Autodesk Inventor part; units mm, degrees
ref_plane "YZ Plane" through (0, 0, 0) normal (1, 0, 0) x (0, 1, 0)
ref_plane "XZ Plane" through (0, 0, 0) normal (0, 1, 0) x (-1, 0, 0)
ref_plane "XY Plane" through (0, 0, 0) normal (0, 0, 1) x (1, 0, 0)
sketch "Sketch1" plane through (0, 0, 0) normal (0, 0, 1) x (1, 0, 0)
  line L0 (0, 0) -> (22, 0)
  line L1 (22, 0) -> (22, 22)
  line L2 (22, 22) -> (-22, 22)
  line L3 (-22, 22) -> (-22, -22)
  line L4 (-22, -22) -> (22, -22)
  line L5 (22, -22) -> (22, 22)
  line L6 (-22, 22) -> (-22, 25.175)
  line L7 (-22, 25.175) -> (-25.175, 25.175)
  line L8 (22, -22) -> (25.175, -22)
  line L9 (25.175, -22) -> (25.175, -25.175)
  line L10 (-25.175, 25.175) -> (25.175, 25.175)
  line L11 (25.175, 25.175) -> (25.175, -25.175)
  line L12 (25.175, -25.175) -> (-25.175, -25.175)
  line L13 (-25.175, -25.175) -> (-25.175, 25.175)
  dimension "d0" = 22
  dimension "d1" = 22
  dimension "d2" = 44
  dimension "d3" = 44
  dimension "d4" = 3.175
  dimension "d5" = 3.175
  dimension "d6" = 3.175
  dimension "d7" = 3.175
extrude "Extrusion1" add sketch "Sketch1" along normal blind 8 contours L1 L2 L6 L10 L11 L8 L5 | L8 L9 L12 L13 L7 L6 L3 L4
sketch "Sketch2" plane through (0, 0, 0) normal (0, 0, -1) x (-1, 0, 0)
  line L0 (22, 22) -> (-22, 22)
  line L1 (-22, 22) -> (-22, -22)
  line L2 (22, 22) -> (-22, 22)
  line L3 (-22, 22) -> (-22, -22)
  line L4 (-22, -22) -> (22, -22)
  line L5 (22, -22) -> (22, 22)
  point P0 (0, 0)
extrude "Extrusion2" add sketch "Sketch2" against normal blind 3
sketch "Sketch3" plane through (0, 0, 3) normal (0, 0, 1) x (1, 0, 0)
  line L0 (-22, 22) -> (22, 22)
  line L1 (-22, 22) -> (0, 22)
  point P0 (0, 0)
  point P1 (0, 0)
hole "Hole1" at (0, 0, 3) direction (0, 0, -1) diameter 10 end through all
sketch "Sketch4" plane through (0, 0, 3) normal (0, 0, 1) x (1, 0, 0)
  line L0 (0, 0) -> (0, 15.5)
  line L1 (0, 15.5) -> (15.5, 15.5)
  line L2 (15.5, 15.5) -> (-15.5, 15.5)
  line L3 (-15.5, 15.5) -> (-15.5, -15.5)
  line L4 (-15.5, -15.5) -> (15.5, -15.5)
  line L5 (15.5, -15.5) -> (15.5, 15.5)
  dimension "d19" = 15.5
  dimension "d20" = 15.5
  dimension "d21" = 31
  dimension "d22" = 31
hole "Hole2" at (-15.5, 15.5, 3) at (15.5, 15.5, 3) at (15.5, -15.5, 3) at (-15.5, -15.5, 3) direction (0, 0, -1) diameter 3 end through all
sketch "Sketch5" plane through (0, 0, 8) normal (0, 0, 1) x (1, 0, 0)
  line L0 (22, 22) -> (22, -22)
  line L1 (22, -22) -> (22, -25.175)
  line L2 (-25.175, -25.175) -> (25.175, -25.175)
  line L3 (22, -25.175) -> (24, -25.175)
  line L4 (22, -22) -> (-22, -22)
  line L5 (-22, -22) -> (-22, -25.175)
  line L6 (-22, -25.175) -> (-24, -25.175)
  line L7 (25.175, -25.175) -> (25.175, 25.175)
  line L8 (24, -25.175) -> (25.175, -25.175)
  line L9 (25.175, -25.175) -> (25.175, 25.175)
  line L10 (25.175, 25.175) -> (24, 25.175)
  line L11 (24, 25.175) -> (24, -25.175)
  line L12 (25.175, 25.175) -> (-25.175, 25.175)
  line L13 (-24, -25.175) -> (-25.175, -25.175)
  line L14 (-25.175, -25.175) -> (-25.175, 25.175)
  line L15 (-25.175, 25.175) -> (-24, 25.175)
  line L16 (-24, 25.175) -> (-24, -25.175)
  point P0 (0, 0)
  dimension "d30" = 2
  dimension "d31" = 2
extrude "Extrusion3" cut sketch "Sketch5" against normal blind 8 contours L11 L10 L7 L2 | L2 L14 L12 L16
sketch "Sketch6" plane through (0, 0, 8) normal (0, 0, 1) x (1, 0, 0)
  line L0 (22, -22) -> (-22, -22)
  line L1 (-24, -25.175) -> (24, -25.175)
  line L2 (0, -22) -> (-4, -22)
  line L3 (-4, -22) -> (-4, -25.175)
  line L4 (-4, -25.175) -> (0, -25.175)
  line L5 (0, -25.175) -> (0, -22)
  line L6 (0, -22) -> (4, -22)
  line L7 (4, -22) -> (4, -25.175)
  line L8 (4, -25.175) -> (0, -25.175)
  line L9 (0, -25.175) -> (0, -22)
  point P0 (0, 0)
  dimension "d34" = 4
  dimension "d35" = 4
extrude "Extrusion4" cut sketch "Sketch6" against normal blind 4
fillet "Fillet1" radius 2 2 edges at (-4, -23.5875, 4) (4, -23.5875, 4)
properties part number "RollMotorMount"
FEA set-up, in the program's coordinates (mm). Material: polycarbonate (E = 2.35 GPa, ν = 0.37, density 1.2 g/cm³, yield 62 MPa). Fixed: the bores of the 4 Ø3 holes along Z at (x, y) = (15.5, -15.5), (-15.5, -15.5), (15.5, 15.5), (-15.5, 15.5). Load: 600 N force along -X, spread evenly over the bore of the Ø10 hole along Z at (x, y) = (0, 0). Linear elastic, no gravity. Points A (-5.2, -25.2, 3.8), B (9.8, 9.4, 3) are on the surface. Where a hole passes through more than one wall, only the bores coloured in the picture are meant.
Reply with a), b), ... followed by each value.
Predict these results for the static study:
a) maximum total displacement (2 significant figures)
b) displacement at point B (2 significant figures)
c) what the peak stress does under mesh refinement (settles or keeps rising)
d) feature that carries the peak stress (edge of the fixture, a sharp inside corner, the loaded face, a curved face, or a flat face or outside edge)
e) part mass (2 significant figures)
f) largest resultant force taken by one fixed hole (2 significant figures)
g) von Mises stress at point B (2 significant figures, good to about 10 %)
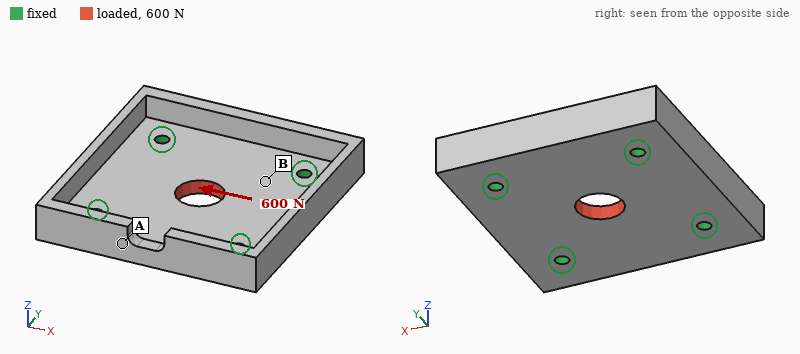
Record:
a) 52 µm
b) 22 µm
c) keeps rising
d) edge of the fixture
e) 11 g
f) 160 N
g) 5.1 MPa
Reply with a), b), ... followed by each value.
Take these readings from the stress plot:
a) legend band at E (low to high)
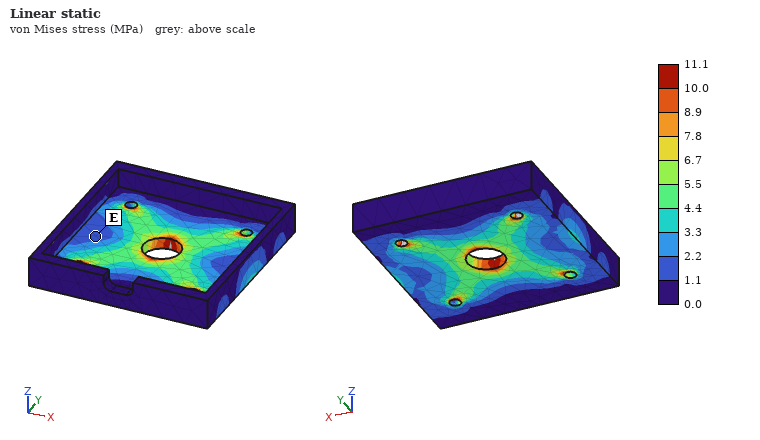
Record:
a) 1.1 to 2.2 MPa
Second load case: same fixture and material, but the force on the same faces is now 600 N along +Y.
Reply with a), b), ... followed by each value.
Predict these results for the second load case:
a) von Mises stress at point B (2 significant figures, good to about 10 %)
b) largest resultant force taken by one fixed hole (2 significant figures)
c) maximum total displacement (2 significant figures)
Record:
a) 4.9 MPa
b) 160 N
c) 51 µm
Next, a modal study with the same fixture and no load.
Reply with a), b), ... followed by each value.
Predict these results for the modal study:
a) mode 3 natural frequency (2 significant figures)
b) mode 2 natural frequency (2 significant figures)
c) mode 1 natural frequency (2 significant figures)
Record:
a) 3700 Hz
b) 3300 Hz
c) 3300 Hz
